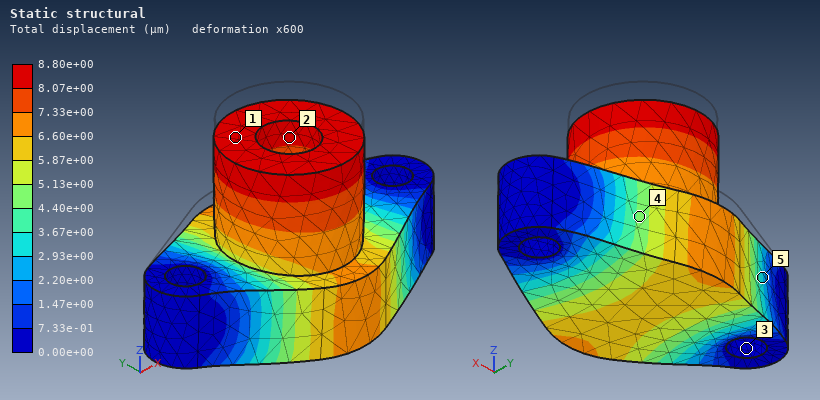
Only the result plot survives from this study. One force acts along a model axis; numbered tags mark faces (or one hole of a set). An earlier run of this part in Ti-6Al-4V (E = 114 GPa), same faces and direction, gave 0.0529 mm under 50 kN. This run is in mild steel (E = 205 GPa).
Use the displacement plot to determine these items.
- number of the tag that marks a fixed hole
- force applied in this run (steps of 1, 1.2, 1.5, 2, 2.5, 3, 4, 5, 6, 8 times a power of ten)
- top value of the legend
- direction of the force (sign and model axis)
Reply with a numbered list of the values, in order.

1. 3
2. 15 kN
3. 8.80e+00 µm
4. -Z
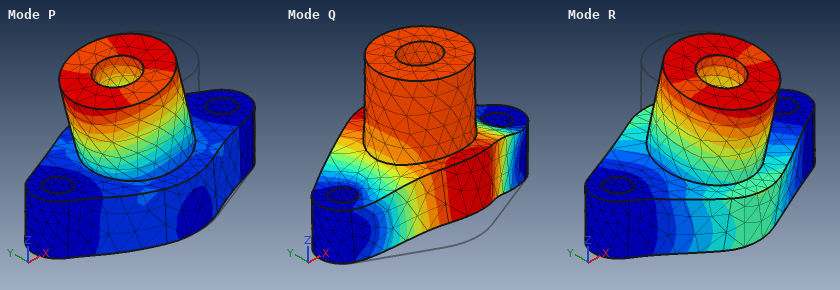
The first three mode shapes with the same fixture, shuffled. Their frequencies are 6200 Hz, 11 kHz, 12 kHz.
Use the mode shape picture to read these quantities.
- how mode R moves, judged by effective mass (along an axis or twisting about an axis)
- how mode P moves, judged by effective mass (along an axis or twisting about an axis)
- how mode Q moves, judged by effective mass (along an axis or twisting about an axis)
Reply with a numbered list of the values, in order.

1. along Y
2. along X
3. along Z
